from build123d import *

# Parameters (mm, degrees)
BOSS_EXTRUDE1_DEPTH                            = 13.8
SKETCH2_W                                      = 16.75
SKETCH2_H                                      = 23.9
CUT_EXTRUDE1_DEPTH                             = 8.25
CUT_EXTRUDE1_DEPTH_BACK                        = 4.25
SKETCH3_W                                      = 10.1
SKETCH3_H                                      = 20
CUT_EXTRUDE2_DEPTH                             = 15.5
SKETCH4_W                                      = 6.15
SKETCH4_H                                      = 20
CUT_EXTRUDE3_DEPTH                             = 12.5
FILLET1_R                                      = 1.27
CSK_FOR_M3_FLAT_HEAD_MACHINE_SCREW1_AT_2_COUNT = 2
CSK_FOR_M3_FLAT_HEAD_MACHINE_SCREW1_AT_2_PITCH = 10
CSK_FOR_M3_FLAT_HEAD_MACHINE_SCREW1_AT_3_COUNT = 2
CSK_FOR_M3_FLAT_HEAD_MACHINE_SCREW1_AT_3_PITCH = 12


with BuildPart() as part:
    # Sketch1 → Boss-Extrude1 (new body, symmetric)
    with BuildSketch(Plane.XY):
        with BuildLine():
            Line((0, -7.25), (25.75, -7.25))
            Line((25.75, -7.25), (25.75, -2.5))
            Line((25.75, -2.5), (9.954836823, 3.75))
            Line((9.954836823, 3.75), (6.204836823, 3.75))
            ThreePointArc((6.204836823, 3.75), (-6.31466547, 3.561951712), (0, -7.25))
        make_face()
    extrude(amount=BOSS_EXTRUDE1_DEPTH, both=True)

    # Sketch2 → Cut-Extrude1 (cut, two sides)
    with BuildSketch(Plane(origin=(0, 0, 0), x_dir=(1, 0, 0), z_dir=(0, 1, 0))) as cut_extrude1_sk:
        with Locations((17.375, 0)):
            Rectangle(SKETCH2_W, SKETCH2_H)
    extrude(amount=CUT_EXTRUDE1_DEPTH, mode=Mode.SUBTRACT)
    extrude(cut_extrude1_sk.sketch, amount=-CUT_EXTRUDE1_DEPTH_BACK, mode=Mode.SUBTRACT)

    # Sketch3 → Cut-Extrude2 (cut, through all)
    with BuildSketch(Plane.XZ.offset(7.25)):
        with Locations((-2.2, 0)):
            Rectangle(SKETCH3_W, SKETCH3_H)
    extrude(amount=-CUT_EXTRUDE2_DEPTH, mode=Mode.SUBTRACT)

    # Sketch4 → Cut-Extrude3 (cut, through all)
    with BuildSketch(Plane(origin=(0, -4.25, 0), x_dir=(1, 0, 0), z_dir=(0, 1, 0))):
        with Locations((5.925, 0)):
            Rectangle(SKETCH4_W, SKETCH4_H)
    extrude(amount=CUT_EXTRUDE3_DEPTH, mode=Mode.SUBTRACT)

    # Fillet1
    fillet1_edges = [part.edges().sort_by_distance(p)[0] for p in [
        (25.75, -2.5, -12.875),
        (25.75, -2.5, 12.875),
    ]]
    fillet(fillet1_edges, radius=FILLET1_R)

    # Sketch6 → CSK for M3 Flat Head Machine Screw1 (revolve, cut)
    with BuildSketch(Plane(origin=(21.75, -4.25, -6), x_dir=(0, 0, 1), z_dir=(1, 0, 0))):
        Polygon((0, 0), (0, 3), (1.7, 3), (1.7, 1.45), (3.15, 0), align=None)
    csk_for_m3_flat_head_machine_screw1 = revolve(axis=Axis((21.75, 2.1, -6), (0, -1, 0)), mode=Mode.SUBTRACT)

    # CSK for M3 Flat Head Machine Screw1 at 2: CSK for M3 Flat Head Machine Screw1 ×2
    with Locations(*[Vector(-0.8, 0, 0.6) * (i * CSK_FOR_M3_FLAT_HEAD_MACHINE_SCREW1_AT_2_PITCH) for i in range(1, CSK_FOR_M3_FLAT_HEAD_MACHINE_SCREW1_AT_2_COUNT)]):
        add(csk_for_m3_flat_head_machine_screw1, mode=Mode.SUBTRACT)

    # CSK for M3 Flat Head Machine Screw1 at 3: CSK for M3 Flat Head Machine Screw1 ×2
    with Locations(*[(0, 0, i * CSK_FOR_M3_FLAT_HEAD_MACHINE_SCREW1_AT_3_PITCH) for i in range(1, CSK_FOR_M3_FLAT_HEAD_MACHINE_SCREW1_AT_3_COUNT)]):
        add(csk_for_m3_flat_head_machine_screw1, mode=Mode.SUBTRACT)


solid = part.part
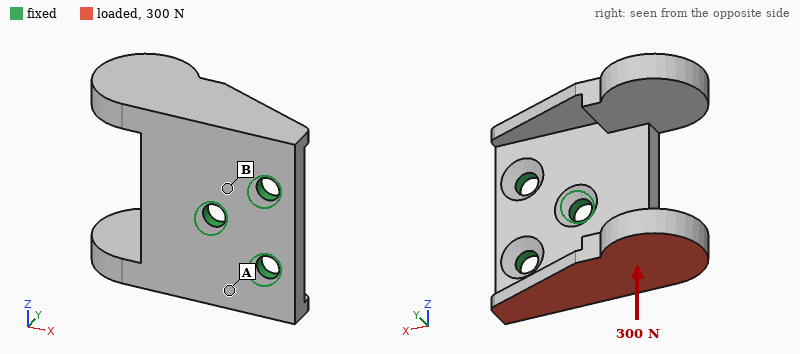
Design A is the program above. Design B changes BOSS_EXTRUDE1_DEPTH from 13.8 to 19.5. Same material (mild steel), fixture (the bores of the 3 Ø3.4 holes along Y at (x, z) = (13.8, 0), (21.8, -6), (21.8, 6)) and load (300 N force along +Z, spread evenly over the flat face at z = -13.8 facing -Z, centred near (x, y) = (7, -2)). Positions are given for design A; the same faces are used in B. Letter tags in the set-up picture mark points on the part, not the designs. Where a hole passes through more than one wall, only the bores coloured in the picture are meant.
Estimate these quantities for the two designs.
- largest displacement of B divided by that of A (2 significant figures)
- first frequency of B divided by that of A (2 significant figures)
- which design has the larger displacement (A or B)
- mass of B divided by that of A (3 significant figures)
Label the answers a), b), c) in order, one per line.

a) 0.75
b) 0.62
c) A
d) 2.10
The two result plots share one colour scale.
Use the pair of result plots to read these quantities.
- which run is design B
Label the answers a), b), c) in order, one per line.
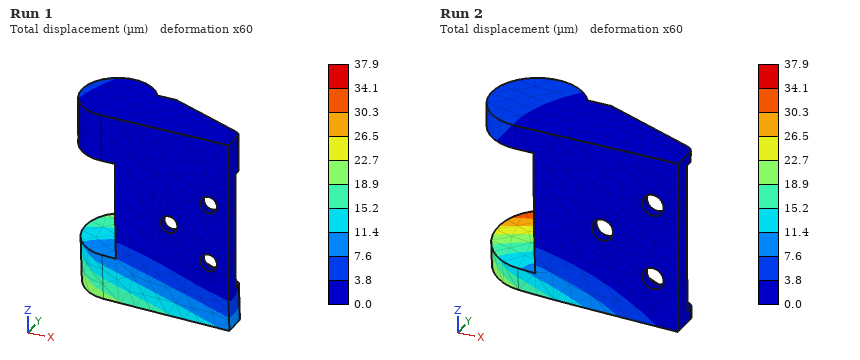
a) Run 1
